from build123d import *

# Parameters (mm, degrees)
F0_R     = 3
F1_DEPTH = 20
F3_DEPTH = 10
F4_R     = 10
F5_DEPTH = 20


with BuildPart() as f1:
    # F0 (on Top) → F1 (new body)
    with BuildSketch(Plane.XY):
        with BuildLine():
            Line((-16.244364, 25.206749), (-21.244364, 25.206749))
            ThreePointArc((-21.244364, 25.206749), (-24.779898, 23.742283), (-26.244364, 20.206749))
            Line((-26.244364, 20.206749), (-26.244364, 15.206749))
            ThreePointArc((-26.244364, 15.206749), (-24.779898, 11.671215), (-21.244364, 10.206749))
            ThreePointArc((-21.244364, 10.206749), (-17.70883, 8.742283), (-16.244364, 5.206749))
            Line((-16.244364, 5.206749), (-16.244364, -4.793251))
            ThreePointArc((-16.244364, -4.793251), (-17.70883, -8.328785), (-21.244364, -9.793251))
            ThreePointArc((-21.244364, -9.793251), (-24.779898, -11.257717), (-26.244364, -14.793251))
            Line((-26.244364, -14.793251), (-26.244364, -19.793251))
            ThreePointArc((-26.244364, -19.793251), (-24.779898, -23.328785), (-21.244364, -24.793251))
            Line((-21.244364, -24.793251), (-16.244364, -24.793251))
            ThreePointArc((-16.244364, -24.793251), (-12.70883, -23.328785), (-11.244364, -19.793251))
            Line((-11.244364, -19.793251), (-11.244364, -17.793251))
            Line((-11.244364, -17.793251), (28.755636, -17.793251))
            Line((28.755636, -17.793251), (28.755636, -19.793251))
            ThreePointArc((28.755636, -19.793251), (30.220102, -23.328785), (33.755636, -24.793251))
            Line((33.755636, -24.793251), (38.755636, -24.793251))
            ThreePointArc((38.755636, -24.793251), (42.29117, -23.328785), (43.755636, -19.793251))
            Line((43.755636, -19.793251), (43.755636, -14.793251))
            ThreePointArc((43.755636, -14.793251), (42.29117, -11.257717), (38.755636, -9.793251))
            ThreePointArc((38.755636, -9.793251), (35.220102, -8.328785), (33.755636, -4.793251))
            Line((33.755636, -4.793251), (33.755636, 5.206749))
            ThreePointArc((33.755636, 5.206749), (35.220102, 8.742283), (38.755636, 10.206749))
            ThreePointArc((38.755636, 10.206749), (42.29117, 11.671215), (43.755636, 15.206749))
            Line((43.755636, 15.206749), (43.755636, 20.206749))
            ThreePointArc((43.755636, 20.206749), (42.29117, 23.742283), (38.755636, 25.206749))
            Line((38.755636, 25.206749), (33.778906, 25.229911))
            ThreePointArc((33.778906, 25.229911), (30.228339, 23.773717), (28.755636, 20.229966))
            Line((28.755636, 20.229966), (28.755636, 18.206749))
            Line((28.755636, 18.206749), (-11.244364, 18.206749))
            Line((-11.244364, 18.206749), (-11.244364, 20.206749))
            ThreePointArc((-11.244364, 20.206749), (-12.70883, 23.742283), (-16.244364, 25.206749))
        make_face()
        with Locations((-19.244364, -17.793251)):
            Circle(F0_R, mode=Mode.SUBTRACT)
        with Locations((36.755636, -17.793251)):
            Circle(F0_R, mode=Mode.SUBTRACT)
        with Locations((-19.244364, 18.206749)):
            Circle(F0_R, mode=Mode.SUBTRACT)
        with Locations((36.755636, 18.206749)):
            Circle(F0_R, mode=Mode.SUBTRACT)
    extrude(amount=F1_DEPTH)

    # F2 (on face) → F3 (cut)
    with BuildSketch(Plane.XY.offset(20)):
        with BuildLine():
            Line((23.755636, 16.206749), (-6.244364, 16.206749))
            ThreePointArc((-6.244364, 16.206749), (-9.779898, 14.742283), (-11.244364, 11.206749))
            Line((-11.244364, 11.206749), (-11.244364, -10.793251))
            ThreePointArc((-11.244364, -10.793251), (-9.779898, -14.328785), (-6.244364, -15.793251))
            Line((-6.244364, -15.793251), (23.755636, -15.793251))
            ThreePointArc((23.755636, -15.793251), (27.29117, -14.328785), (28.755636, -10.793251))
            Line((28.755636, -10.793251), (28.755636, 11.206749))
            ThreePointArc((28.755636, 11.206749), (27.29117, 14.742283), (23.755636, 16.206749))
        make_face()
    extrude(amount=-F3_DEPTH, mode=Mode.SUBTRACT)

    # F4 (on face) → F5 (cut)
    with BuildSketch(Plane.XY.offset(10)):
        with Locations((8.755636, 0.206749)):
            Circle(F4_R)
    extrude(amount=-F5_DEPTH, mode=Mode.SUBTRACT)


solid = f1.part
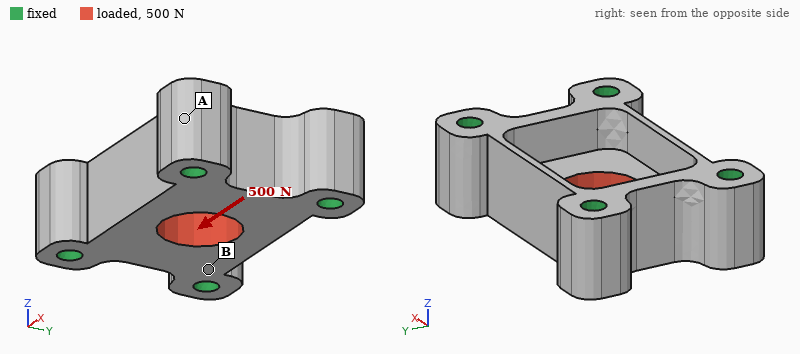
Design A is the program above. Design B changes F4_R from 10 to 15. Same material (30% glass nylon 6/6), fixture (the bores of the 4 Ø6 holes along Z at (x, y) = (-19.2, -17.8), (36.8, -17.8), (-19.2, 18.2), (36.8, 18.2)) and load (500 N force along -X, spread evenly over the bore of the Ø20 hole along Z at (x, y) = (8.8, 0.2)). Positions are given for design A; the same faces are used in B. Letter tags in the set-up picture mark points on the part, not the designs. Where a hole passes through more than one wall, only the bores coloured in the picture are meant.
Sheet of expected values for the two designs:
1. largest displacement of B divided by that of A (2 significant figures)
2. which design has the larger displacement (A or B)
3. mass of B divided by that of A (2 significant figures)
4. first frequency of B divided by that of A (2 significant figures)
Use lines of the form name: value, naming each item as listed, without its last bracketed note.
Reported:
largest displacement of B divided by that of A: 1.1
which design has the larger displacement: B
mass of B divided by that of A: 0.88
first frequency of B divided by that of A: 0.88
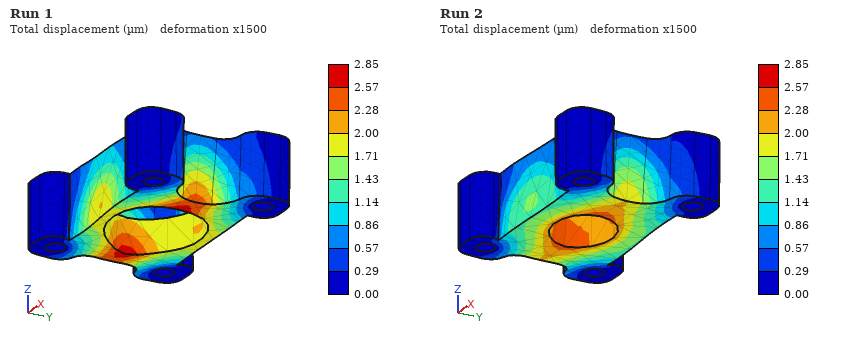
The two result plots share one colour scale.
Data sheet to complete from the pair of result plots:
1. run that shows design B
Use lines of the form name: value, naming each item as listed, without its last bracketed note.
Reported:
run that shows design B: Run 1
